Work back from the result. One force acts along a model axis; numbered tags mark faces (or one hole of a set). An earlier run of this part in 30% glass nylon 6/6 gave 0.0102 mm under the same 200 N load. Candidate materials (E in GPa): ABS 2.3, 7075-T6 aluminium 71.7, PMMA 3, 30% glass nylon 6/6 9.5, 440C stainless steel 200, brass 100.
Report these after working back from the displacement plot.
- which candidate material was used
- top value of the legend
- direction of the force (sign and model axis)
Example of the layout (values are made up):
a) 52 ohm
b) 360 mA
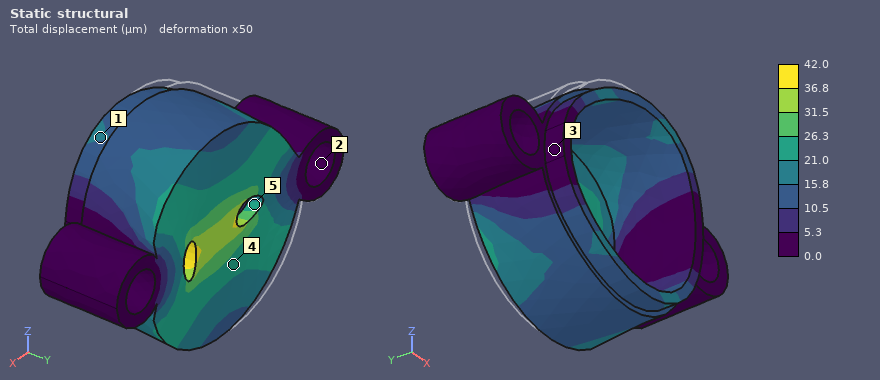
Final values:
a) ABS
b) 42.0 µm
c) +X
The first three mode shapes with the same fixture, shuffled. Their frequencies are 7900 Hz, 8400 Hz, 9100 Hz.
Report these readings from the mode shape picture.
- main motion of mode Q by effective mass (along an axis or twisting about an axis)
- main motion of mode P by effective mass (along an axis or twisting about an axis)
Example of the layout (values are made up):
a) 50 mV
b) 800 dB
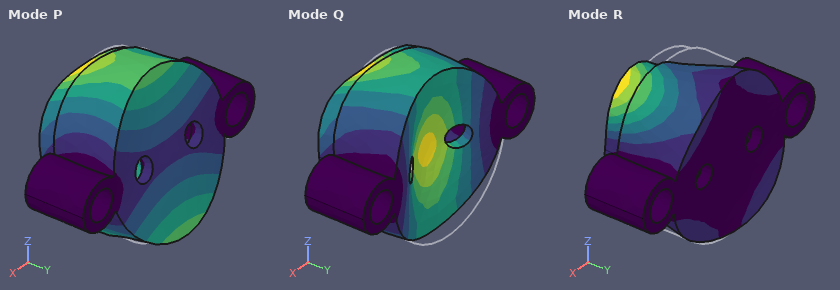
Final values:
a) along Y
b) twisting about X
